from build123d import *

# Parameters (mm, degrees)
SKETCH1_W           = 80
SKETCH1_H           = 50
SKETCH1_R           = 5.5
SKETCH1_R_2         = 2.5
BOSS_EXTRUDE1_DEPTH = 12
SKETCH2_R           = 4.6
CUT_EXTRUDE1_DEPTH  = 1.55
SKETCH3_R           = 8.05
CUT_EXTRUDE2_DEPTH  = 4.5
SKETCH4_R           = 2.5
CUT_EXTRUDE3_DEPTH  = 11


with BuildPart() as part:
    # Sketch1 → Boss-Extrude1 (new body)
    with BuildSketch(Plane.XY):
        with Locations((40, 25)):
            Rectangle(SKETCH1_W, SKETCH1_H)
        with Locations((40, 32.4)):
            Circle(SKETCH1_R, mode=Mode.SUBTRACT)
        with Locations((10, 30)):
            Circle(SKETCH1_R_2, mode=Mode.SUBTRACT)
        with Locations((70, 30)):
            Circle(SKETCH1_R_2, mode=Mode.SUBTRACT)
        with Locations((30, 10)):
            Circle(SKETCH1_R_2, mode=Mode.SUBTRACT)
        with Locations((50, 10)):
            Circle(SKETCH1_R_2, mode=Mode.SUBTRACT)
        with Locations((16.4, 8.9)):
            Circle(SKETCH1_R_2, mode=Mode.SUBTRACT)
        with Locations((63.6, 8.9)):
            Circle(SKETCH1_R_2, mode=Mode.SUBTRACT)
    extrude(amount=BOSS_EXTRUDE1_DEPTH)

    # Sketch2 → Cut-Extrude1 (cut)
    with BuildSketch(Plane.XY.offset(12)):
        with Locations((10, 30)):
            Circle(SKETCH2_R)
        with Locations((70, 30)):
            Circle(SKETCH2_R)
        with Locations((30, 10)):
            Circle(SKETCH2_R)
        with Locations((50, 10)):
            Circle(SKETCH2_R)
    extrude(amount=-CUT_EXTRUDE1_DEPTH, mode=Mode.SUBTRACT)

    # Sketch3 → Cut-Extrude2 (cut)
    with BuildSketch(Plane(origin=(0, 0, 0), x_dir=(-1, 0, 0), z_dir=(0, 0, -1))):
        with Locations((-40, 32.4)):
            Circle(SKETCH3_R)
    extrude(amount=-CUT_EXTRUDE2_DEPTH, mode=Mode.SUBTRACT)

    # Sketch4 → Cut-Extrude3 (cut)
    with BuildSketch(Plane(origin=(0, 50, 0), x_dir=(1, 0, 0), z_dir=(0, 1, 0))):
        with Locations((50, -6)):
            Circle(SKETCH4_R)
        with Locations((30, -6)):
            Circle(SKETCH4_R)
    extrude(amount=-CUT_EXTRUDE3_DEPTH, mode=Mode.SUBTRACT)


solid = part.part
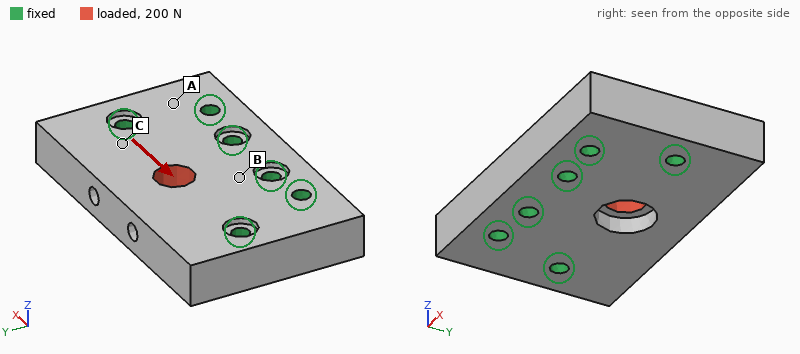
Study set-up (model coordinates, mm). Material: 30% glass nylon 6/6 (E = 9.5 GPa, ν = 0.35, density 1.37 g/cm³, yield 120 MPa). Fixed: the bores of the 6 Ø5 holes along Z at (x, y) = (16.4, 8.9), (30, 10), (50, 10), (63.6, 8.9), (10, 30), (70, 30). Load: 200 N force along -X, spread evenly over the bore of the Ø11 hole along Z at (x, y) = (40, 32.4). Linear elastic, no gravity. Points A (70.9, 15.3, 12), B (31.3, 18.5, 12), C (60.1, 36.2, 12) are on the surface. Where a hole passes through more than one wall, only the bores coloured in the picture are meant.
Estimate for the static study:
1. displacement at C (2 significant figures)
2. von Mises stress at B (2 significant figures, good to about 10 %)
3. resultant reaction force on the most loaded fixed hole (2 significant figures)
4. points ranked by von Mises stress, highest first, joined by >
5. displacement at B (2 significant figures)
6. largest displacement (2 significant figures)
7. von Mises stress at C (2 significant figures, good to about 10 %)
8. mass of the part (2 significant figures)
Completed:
0.64 µm
0.26 MPa
71 N
C > B > A
0.29 µm
1.7 µm
0.41 MPa
61 g
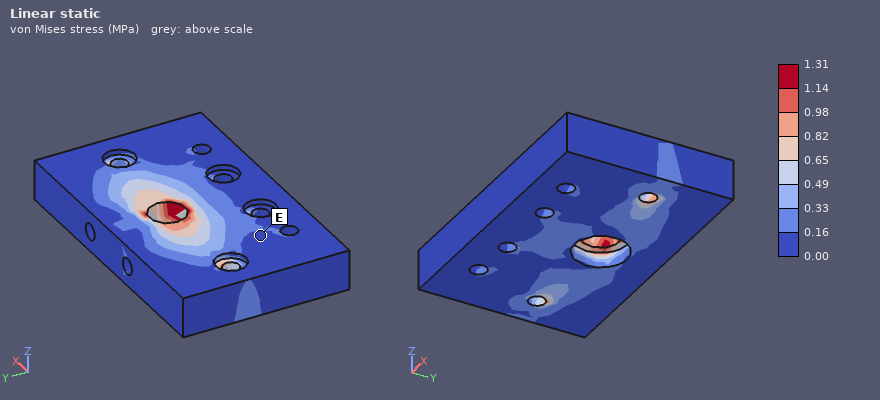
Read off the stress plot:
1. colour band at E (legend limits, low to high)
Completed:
0.00 to 0.16 MPa
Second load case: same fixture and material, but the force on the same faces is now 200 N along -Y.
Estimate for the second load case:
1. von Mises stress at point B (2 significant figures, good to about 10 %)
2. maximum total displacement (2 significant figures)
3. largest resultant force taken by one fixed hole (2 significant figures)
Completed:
0.53 MPa
2.7 µm
65 N
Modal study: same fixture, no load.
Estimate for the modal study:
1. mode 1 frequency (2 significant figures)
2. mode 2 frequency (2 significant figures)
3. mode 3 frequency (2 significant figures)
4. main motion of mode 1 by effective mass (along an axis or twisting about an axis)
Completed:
6000 Hz
9500 Hz
11 kHz
along Z
